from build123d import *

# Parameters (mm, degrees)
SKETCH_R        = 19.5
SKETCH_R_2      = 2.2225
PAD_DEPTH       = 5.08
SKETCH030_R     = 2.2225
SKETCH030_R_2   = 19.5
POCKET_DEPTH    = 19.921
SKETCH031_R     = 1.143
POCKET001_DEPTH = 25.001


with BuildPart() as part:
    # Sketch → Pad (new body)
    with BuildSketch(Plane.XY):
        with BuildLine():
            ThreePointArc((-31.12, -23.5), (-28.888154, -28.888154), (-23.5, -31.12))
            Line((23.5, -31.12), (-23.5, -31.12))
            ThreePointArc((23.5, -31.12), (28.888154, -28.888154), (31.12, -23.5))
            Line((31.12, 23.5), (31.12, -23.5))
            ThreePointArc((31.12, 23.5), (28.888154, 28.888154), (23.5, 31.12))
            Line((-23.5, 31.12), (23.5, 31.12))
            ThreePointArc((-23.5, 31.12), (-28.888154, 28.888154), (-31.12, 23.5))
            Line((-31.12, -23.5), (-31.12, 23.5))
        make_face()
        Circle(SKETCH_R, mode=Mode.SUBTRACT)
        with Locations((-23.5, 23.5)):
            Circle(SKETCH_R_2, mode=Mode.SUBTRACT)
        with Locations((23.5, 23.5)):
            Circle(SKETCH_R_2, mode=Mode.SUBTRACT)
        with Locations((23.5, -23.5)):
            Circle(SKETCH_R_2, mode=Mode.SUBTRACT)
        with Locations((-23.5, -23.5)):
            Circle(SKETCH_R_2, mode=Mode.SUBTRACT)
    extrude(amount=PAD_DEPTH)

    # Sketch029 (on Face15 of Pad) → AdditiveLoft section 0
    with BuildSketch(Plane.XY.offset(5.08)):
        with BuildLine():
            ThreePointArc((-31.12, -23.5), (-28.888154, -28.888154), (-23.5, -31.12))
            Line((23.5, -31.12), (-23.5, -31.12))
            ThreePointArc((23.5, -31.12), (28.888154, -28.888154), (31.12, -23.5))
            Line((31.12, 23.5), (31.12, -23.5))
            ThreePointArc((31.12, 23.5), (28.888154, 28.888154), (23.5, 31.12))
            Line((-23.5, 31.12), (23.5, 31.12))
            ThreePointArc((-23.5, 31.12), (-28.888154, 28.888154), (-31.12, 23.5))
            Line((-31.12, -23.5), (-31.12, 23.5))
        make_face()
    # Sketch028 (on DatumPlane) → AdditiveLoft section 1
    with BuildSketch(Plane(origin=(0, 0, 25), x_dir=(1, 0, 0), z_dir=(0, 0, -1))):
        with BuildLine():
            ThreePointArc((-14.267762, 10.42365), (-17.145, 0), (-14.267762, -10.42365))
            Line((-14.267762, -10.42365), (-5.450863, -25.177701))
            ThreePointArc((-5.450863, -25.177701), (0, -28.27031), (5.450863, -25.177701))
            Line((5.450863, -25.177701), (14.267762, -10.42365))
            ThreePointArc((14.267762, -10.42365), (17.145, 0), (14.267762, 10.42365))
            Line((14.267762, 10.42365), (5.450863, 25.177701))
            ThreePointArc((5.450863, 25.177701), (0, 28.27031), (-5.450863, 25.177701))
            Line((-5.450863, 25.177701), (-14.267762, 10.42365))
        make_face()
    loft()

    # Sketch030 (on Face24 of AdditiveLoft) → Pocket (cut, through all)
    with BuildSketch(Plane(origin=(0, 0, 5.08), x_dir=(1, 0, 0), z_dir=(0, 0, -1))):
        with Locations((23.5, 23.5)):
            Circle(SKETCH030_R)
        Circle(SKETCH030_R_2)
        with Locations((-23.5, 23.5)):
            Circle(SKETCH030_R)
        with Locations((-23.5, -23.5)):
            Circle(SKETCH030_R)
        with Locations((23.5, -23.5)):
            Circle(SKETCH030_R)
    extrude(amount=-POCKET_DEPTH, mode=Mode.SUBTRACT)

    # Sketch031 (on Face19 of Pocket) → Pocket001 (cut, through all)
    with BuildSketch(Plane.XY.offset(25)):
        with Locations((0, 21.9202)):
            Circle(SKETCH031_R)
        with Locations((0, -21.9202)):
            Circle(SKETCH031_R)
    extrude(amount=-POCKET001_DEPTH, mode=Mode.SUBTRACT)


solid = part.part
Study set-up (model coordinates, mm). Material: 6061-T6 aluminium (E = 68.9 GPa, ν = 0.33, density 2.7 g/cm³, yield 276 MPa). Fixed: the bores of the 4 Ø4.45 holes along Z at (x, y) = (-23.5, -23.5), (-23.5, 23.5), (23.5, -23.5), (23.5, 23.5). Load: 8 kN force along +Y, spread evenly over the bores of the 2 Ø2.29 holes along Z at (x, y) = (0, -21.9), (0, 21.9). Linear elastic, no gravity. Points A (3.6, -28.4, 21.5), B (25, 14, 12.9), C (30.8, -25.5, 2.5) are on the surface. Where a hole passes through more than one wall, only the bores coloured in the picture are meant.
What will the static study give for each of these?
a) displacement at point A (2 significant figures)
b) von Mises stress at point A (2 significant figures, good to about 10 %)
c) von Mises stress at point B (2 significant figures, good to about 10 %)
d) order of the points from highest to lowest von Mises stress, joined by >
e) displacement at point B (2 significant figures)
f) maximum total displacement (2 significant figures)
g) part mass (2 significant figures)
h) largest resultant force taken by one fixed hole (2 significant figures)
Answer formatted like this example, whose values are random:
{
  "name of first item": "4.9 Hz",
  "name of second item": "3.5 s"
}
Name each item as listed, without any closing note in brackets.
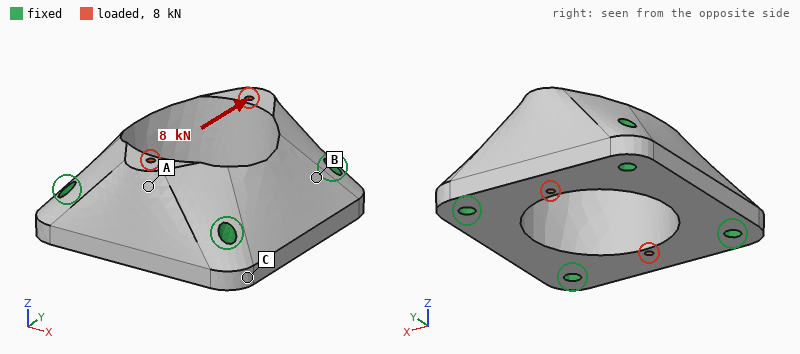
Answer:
{
  "displacement at point A": "18 µm",
  "von Mises stress at point A": "29 MPa",
  "von Mises stress at point B": "18 MPa",
  "order of the points from highest to lowest von Mises stress, joined by >": "A > B > C",
  "displacement at point B": "4.1 µm",
  "maximum total displacement": "23 µm",
  "part mass": "110 g",
  "largest resultant force taken by one fixed hole": "2.1 kN"
}
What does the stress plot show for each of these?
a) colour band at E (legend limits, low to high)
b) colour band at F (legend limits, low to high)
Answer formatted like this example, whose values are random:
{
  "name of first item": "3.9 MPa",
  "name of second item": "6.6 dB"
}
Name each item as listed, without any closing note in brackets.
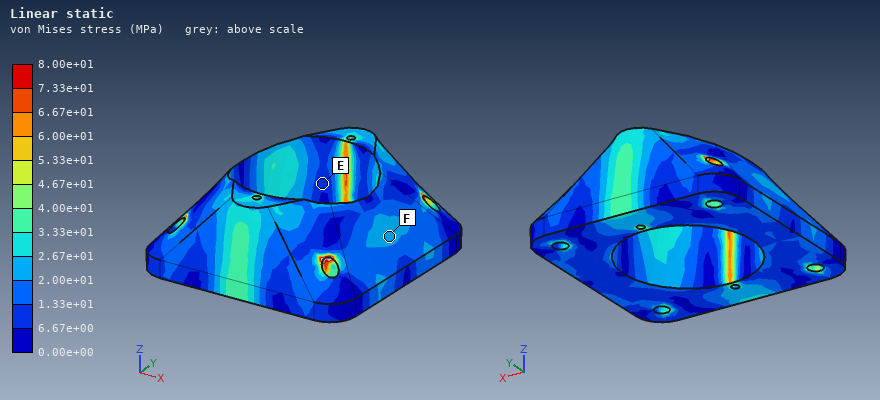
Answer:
{
  "colour band at E": "6.67e+00 to 1.33e+01 MPa",
  "colour band at F": "2.00e+01 to 2.67e+01 MPa"
}
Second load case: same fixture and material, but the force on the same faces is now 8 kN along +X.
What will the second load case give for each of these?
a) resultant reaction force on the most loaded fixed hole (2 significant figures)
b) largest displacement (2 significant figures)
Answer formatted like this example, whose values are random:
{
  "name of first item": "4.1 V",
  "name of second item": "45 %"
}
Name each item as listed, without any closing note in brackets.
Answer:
{
  "resultant reaction force on the most loaded fixed hole": "2.1 kN",
  "largest displacement": "5.4 µm"
}
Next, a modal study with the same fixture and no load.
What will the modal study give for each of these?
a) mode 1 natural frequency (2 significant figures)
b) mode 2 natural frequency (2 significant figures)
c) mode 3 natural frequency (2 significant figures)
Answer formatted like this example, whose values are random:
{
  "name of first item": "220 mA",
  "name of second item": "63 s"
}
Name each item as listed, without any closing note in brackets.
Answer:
{
  "mode 1 natural frequency": "14 kHz",
  "mode 2 natural frequency": "20 kHz",
  "mode 3 natural frequency": "20 kHz"
}
